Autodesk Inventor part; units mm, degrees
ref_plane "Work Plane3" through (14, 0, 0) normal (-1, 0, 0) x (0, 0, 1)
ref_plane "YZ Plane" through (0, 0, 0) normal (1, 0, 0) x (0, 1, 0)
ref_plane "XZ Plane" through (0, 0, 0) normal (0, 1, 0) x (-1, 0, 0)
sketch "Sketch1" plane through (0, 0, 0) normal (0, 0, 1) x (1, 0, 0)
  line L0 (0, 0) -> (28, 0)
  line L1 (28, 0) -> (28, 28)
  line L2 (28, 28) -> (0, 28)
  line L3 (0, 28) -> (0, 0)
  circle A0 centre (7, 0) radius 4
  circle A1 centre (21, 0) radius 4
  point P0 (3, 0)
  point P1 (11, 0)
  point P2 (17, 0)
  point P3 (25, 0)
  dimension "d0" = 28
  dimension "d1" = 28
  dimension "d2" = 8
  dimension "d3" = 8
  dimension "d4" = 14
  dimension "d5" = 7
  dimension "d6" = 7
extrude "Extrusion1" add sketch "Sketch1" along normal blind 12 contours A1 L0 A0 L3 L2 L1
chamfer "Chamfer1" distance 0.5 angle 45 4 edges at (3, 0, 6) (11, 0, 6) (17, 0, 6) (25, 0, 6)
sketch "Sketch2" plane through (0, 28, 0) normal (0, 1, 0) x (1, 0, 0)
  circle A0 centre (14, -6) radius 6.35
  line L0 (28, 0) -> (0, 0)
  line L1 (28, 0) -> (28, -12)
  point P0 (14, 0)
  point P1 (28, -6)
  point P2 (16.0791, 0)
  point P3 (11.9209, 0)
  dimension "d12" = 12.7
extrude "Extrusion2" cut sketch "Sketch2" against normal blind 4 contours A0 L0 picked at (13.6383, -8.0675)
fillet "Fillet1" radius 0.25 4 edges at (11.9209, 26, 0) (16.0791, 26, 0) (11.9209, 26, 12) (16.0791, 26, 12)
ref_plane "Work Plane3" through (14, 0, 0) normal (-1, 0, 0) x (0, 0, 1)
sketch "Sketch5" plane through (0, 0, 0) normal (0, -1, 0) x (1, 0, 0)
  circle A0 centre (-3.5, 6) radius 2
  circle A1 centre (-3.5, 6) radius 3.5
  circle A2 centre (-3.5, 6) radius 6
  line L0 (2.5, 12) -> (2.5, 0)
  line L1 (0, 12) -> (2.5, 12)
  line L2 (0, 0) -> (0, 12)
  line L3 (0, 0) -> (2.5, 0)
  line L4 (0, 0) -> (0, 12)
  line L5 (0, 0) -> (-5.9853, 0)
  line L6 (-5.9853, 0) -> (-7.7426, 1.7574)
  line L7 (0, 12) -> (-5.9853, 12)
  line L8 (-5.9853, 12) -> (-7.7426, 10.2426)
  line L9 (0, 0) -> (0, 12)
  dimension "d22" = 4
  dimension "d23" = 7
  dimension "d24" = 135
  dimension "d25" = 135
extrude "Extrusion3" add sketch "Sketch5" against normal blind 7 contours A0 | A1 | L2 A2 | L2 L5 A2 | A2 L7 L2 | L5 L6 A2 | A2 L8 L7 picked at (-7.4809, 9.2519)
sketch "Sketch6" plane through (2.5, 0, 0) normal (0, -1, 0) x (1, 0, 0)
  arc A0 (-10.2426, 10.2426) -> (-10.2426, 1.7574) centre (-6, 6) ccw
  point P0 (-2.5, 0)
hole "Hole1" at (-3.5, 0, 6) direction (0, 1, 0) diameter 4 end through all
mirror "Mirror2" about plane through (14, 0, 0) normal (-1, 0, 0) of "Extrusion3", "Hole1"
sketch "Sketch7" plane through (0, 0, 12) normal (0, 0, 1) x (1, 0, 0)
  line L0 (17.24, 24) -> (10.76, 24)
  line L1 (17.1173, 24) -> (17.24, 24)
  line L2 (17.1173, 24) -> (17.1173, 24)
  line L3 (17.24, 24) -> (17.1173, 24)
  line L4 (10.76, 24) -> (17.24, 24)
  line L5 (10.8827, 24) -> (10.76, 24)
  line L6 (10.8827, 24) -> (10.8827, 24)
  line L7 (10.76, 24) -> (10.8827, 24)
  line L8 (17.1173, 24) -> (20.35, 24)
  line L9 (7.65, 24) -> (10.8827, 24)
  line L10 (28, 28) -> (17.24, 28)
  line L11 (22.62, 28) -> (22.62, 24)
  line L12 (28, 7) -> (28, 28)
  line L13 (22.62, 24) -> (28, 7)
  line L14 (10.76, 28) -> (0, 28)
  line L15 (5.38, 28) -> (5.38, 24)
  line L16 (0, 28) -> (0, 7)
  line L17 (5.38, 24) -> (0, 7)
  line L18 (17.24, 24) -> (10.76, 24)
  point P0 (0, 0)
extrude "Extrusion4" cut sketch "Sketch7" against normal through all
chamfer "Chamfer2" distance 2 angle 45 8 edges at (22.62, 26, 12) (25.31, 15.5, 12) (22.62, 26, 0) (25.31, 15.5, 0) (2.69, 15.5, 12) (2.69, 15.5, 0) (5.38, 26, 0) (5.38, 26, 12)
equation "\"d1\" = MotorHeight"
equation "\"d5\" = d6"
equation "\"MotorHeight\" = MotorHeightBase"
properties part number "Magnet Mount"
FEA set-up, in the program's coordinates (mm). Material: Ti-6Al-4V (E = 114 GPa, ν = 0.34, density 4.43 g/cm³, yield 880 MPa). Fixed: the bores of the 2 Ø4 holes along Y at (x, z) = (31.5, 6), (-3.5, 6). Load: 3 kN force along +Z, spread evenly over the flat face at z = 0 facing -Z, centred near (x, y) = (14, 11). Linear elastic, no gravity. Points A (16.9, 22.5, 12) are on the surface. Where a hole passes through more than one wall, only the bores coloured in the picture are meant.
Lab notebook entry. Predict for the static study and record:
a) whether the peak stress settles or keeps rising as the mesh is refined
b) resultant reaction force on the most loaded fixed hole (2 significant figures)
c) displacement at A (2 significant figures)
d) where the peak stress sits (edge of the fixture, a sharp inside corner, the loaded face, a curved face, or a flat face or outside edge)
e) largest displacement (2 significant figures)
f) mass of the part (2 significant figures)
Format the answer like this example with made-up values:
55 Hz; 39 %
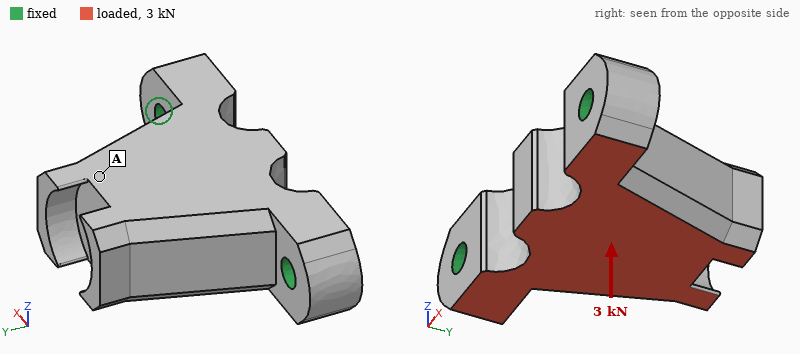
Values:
keeps rising; 1.5 kN; 46 µm; edge of the fixture; 60 µm; 34 g
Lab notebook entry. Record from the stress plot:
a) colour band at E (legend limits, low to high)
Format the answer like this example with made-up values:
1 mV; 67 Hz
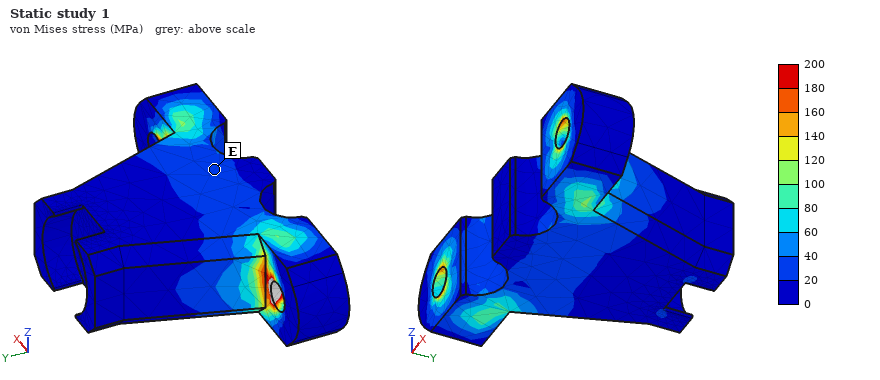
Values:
20 to 40 MPa
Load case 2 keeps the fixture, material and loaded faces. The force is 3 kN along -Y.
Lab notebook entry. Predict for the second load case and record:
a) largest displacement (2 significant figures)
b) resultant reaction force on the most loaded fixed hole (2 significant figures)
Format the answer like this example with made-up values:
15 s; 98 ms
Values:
43 µm; 1.7 kN
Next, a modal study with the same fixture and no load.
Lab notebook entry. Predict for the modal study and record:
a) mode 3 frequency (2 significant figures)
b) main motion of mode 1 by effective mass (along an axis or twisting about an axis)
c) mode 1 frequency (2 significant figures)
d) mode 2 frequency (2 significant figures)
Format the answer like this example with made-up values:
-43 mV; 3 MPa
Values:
24 kHz; along Z; 7800 Hz; 23 kHz
